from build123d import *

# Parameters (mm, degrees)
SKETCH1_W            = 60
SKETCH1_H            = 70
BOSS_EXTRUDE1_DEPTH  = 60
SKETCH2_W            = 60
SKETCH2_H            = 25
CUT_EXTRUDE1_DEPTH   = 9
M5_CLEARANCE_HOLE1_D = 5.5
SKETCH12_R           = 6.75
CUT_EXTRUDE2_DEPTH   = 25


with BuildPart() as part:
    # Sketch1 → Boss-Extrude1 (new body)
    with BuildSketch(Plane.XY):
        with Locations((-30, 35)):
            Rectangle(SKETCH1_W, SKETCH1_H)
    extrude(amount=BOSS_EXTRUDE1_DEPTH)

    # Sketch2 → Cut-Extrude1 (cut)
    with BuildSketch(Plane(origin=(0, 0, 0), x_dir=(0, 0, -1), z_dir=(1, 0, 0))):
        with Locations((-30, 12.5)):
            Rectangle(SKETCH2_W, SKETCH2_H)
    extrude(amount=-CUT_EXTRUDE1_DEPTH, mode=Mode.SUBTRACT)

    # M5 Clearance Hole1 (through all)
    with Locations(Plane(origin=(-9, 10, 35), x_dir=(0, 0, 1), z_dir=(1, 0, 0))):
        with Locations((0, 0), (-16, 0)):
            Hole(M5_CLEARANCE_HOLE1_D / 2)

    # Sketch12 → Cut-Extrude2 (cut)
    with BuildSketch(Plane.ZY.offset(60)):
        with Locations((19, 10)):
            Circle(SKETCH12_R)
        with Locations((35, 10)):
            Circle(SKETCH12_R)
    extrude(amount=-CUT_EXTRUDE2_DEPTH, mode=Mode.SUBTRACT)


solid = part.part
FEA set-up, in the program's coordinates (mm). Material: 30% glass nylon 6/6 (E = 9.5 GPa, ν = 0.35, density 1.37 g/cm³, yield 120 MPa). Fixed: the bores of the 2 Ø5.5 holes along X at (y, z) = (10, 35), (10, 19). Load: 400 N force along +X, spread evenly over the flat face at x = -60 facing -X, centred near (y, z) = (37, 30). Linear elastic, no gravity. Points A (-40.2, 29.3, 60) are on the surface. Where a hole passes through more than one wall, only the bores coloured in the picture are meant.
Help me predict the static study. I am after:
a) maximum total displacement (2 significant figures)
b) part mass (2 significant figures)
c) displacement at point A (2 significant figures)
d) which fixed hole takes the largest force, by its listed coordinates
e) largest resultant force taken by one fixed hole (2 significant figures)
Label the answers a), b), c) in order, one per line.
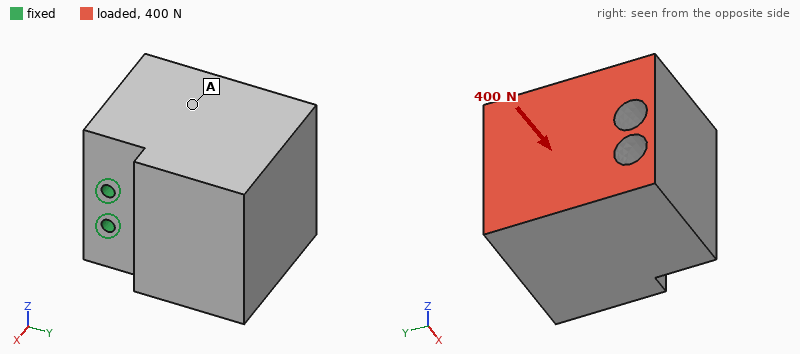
a) 17 µm
b) 320 g
c) 6.7 µm
d) (10, 35)
e) 230 N
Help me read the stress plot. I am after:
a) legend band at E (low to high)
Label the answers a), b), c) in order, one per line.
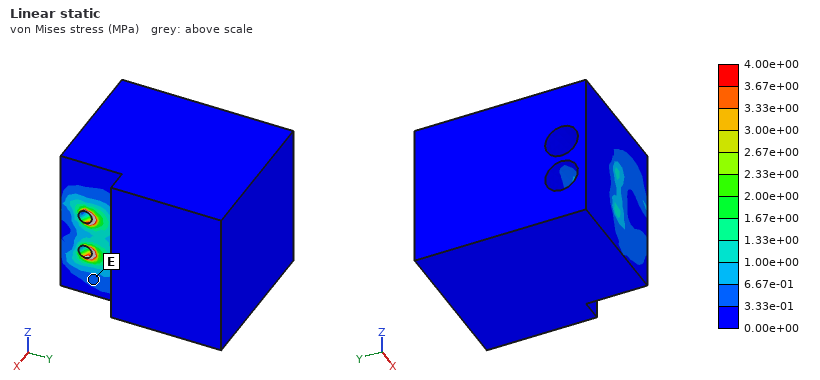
a) 3.33e-01 to 6.67e-01 MPa
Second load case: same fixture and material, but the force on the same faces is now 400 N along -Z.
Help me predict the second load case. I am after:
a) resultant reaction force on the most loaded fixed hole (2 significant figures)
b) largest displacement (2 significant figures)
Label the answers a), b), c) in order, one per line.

a) 650 N
b) 22 µm
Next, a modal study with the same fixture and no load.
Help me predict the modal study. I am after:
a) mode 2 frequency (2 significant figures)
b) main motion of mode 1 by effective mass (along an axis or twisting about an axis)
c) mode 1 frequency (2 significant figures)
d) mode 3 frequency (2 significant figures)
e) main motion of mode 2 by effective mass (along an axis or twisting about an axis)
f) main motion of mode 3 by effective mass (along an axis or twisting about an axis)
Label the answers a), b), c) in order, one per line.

a) 1700 Hz
b) along X
c) 1600 Hz
d) 3100 Hz
e) along Z
f) twisting about Y
